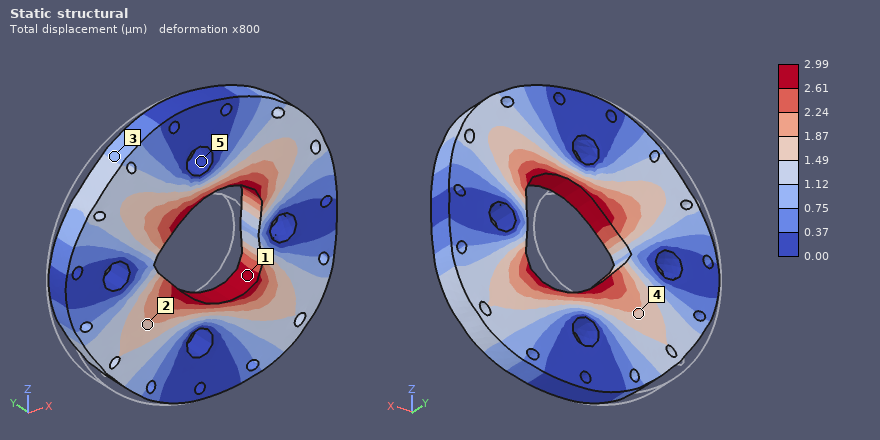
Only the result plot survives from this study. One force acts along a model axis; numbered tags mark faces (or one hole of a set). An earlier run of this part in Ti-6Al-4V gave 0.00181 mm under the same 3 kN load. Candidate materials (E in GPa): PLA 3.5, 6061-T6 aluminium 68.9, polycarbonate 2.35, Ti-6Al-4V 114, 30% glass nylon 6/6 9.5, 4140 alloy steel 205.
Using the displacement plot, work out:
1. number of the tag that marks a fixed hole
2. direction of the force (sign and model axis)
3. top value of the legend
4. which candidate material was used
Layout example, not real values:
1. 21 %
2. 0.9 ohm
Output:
1. 5
2. +X
3. 2.99 µm
4. 6061-T6 aluminium
